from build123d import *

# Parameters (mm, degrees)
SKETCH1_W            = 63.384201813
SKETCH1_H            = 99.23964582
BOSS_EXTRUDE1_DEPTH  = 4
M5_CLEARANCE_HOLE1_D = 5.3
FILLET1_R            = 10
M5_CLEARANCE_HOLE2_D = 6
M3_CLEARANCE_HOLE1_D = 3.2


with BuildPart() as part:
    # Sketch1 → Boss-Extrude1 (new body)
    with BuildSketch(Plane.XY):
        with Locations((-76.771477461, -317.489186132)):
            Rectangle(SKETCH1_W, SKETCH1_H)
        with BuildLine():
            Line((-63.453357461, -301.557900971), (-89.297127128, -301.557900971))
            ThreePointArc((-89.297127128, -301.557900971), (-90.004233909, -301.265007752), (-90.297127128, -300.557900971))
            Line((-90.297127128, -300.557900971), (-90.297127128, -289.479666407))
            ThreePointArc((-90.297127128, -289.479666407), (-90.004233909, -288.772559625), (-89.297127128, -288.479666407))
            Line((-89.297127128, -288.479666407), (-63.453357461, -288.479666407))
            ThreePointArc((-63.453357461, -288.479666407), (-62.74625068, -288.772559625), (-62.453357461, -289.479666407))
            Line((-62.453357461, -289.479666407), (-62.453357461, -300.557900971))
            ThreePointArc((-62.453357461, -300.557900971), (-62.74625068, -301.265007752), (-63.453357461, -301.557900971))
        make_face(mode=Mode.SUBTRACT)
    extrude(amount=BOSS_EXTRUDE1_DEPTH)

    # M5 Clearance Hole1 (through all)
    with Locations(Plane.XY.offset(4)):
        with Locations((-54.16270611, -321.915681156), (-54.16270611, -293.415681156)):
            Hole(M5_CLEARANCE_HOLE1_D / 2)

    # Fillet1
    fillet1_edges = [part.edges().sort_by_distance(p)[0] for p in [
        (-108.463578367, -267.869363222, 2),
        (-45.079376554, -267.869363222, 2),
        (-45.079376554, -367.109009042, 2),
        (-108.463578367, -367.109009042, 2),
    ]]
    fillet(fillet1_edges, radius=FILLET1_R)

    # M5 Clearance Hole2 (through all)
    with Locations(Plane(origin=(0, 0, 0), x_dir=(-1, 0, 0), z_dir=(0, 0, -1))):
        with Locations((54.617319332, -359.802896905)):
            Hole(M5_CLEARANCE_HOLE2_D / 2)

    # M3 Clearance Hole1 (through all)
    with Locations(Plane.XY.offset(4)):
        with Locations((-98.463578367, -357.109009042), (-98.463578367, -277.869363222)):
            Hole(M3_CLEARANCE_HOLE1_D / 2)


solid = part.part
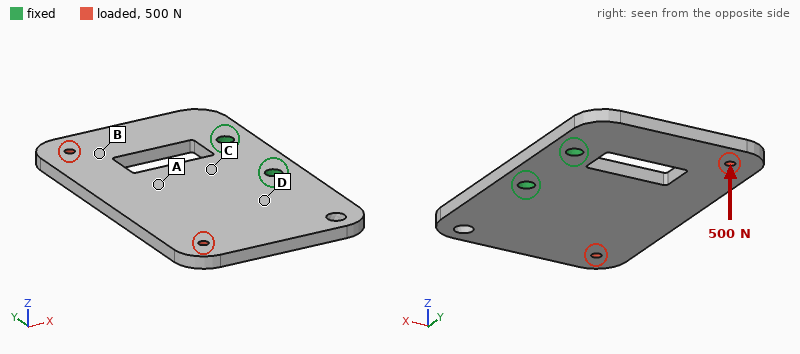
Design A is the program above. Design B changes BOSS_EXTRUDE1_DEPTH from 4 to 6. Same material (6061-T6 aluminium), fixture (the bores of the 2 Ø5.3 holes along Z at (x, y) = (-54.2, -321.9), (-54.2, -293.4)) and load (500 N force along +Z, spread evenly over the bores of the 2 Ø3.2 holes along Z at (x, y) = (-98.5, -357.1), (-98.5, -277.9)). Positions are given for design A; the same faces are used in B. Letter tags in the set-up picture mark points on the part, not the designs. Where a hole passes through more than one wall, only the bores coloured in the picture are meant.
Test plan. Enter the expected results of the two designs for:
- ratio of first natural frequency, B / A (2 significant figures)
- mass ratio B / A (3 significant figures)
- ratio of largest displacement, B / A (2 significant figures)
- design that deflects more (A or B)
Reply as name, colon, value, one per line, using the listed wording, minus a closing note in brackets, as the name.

ratio of first natural frequency, B / A: 1.4
mass ratio B / A: 1.50
ratio of largest displacement, B / A: 0.32
design that deflects more: A
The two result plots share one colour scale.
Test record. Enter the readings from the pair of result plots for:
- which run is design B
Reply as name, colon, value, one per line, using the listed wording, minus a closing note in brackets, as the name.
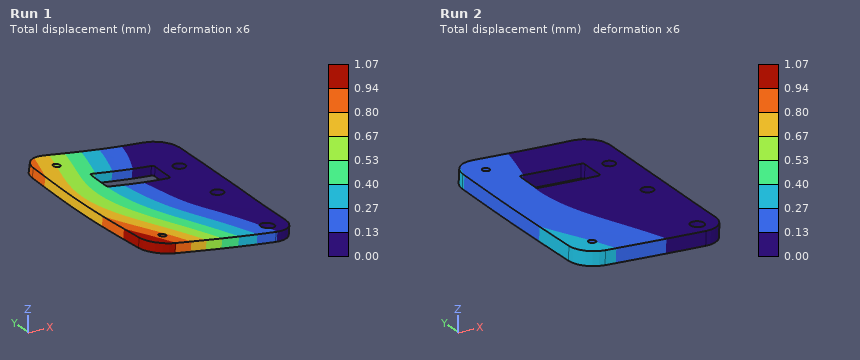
which run is design B: Run 2
